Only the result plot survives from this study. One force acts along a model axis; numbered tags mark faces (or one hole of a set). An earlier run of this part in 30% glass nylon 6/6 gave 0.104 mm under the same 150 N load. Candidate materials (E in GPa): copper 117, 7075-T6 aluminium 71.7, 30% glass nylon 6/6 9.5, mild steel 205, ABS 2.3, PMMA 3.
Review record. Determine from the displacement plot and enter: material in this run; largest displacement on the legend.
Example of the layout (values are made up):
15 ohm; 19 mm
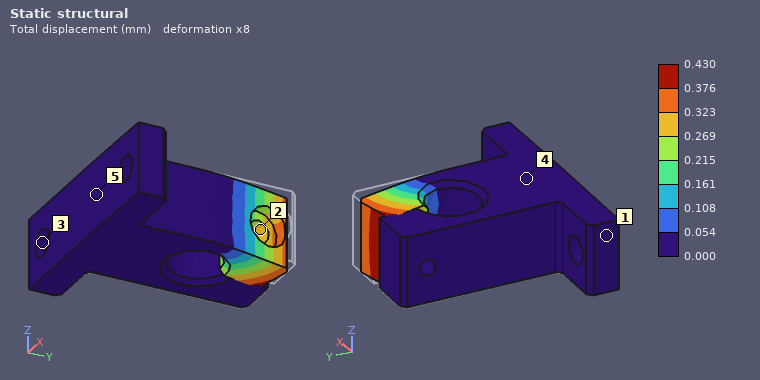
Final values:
ABS; 0.430 mm
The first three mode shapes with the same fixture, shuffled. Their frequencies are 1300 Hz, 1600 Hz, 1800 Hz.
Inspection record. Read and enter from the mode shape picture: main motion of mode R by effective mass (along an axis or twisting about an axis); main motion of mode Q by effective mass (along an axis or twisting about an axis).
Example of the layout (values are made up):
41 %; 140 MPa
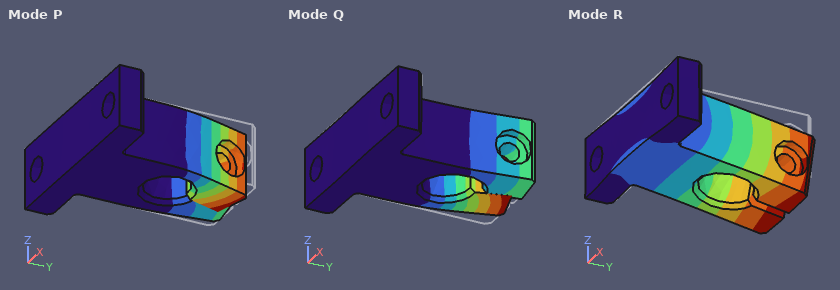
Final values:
along Z; along X
